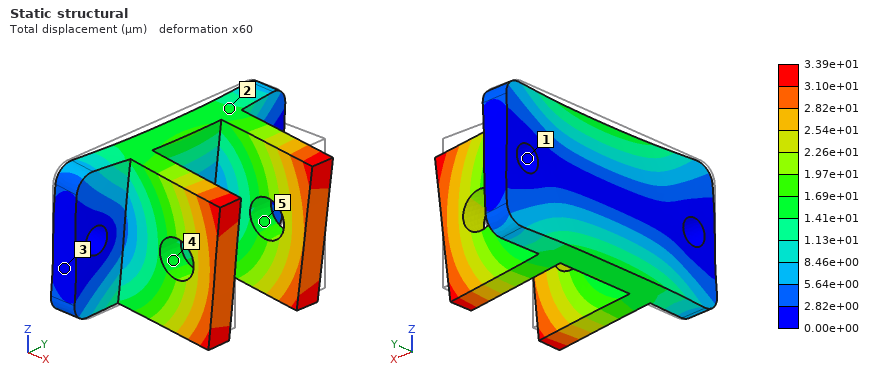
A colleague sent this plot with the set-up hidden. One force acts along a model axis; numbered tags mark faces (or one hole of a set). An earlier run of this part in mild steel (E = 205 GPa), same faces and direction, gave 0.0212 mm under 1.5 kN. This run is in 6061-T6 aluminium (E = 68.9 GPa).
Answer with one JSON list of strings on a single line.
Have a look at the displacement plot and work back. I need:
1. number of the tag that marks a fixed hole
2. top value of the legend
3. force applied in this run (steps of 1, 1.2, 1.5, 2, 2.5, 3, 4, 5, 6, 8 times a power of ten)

["1", "3.39e+01 µm", "800 N"]
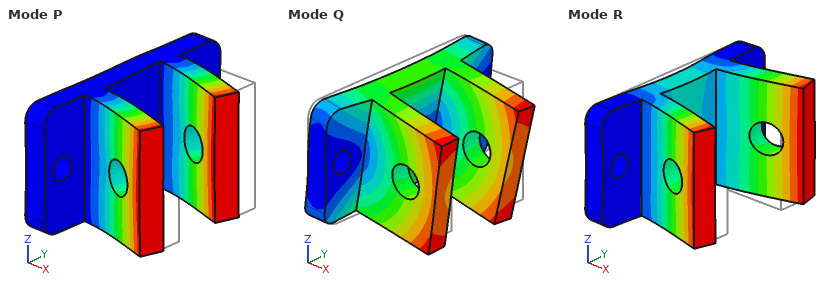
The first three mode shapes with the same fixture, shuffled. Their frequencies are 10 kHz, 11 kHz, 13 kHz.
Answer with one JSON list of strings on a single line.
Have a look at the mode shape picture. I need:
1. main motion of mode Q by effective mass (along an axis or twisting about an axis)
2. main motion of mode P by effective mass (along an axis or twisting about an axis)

["along Z", "along Y"]
